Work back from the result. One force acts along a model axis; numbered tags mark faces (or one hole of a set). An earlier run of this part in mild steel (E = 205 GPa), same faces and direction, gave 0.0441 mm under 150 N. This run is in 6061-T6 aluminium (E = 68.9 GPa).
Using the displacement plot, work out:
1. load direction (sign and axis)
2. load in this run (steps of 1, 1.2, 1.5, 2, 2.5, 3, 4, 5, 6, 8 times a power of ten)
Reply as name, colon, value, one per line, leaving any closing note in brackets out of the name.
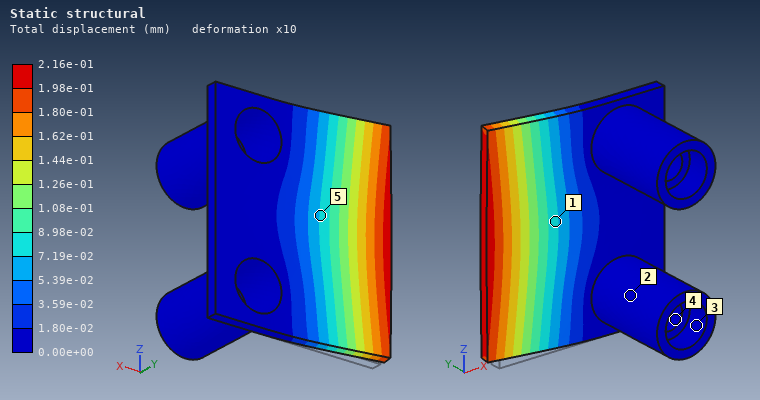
load direction: +Y
load in this run: 250 N
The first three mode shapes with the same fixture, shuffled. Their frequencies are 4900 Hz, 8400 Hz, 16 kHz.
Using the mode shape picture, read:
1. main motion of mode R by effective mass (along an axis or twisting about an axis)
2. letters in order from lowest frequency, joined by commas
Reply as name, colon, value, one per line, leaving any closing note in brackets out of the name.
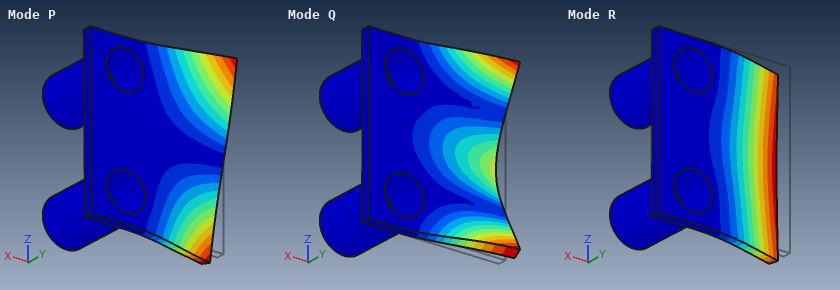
main motion of mode R by effective mass: along Y
letters in order from lowest frequency, joined by commas: R, P, Q
